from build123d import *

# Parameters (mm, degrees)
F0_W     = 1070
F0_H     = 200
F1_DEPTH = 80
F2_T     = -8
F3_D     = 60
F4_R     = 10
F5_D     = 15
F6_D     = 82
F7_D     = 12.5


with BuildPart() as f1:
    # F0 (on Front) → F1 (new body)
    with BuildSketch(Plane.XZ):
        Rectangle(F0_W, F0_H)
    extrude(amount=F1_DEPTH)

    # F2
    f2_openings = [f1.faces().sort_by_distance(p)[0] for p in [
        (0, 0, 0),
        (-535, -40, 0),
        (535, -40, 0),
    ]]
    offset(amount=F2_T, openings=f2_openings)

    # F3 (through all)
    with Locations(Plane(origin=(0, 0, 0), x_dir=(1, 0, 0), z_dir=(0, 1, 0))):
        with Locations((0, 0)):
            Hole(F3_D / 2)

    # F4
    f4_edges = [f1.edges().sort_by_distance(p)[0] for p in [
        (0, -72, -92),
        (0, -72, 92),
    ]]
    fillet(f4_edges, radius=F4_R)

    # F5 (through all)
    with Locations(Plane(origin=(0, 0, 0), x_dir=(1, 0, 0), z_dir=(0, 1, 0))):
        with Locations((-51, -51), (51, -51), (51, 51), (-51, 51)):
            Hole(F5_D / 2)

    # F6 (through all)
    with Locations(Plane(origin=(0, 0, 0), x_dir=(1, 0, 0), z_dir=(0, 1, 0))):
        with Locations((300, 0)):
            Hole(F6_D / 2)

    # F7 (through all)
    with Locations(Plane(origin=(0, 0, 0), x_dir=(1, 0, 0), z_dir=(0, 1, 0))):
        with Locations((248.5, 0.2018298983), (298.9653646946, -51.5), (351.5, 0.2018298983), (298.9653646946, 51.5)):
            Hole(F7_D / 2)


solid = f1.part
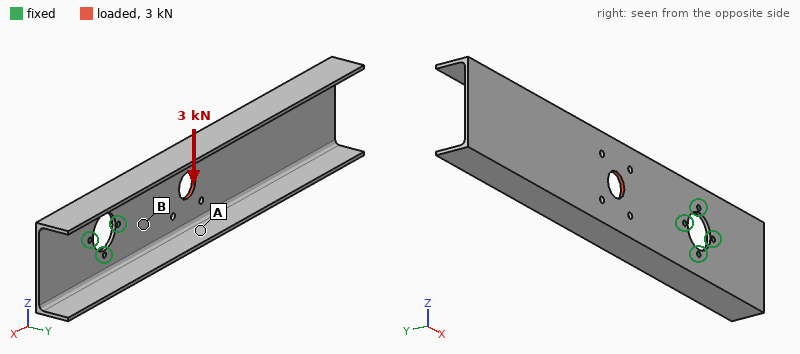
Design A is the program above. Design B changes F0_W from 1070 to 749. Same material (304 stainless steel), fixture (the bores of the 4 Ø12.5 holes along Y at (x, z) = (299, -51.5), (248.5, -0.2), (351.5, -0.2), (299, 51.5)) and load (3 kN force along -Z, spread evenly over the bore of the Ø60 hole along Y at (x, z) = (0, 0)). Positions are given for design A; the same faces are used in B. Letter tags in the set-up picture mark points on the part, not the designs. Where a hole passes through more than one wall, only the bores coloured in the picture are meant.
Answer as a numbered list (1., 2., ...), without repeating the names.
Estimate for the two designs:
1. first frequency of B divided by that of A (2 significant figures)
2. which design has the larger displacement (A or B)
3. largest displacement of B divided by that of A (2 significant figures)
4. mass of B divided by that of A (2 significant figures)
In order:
1. 1.2
2. A
3. 0.76
4. 0.69
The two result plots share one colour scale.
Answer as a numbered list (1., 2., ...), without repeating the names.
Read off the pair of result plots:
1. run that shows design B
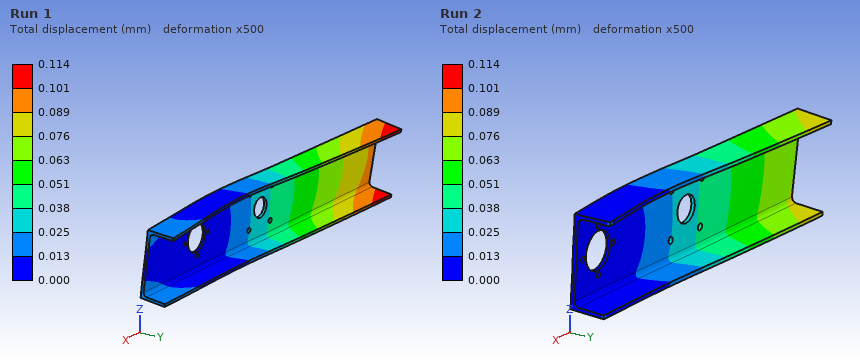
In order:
1. Run 2
